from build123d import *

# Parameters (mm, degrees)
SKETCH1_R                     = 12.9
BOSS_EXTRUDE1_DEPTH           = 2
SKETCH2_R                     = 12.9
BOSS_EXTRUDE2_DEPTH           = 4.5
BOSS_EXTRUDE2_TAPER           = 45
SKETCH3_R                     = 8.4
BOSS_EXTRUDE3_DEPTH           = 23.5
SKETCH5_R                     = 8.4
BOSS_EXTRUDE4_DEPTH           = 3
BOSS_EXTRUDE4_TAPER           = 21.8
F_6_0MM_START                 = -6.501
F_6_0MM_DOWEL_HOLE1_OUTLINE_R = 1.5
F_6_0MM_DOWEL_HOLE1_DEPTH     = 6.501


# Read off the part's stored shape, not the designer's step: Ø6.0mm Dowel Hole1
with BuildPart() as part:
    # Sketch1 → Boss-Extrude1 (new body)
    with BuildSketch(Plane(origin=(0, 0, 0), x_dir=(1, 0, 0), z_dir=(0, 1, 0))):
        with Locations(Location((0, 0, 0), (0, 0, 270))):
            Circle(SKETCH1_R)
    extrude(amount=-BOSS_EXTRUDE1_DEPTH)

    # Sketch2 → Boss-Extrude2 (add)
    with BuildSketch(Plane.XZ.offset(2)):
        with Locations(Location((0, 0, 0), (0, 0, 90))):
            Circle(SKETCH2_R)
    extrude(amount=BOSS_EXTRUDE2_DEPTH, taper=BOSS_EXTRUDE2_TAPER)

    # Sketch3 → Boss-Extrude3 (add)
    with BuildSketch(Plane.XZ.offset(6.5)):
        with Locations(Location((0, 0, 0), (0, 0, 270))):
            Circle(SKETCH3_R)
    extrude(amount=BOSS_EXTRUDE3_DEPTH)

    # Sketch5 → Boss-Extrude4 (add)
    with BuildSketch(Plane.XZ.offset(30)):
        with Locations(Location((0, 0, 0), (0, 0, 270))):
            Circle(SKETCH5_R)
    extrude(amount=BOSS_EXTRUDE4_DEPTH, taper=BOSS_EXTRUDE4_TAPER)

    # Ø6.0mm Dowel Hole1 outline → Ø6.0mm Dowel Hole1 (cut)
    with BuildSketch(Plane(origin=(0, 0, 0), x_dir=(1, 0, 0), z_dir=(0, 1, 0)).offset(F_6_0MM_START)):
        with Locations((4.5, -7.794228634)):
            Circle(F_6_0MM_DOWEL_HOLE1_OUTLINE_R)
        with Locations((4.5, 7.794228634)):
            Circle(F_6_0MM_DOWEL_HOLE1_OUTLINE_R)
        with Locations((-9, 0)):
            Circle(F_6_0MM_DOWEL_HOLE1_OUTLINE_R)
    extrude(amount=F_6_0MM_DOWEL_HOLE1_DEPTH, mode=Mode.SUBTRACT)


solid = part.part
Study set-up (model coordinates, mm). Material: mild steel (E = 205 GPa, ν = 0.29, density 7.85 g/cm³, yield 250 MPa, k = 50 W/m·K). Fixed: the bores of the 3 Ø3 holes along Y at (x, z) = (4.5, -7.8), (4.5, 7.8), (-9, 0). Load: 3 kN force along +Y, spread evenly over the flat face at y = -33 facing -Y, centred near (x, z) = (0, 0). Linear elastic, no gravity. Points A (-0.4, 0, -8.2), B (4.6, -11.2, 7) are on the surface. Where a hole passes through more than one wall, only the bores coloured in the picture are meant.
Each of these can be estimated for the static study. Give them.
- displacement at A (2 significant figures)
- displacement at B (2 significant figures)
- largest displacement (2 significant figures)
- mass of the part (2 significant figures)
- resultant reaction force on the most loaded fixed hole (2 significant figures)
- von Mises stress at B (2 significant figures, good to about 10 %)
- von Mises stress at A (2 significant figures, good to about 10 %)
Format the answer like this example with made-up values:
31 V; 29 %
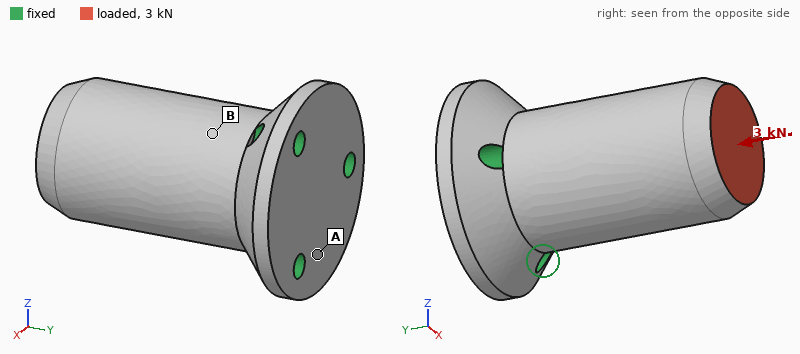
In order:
0.48 µm; 0.89 µm; 2.5 µm; 65 g; 1.0 kN; 17 MPa; 5.8 MPa
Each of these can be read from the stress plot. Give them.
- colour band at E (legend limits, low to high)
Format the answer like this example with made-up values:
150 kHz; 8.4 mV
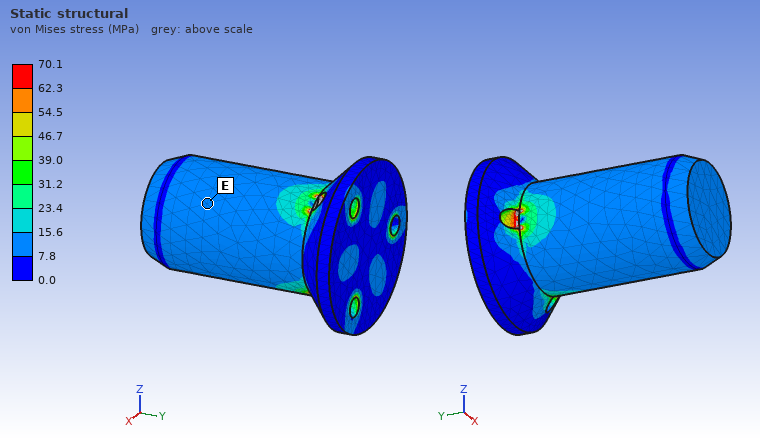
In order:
7.8 to 15.6 MPa
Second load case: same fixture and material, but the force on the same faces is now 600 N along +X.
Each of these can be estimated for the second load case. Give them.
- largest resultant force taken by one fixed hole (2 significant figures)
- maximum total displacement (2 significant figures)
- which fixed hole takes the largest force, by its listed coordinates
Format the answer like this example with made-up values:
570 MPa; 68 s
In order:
1.2 kN; 9.0 µm; (-9, 0)
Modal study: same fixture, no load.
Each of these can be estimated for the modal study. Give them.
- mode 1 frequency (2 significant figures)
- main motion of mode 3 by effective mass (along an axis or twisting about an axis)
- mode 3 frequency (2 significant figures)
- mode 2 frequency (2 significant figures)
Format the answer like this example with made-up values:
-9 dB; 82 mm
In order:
11 kHz; twisting about Y; 29 kHz; 11 kHz
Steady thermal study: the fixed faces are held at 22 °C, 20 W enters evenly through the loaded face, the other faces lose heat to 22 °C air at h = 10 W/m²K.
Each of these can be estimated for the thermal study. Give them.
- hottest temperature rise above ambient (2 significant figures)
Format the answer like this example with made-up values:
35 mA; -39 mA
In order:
57 K
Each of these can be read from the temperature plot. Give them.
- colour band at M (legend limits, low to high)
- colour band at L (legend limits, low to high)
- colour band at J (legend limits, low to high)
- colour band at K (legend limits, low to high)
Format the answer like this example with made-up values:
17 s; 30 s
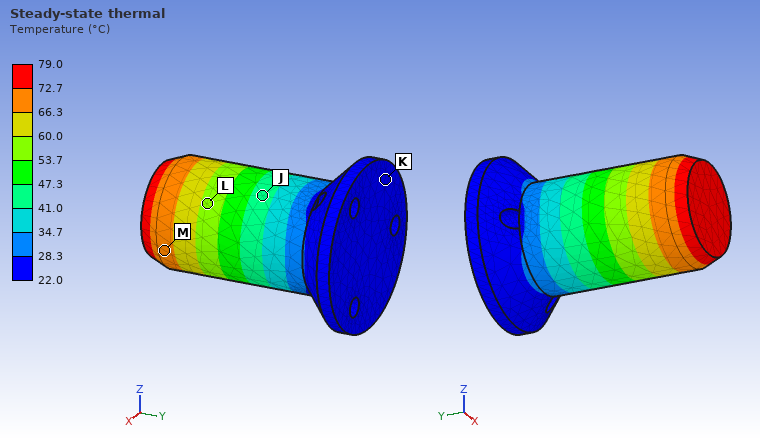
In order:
66.3 to 72.7 °C; 53.7 to 60.0 °C; 41.0 to 47.3 °C; 22.0 to 28.3 °C
